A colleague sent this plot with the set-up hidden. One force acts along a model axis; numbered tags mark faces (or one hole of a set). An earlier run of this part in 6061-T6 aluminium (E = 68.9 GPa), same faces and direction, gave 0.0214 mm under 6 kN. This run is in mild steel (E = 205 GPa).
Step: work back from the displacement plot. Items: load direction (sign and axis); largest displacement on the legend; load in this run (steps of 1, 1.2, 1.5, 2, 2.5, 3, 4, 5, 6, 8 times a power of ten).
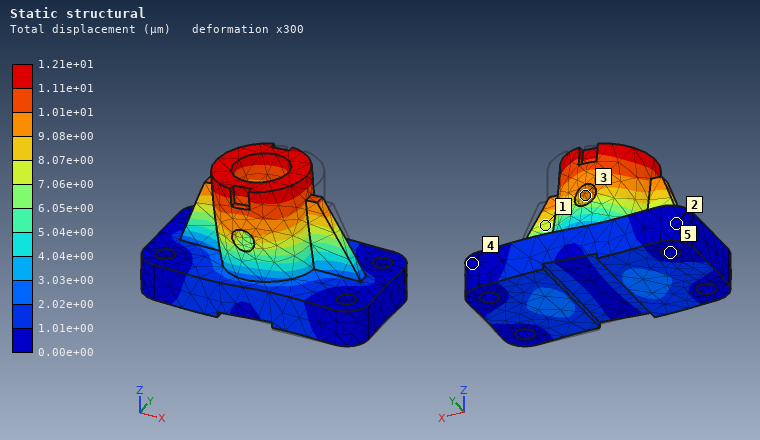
-X
1.21e+01 µm
10 kN
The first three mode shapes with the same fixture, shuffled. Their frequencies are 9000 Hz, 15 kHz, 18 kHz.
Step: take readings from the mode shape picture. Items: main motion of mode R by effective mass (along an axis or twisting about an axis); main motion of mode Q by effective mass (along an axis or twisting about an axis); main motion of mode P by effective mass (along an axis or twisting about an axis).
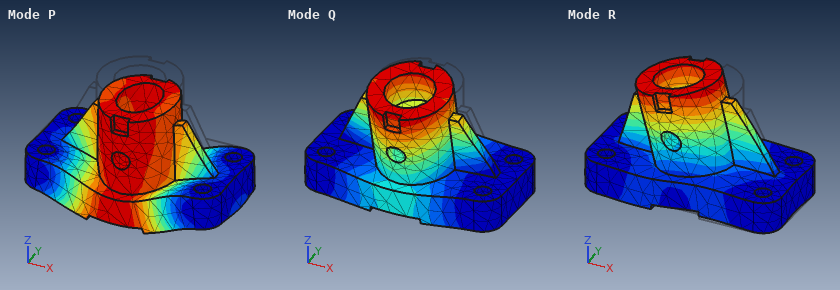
along X
along Y
along Z
